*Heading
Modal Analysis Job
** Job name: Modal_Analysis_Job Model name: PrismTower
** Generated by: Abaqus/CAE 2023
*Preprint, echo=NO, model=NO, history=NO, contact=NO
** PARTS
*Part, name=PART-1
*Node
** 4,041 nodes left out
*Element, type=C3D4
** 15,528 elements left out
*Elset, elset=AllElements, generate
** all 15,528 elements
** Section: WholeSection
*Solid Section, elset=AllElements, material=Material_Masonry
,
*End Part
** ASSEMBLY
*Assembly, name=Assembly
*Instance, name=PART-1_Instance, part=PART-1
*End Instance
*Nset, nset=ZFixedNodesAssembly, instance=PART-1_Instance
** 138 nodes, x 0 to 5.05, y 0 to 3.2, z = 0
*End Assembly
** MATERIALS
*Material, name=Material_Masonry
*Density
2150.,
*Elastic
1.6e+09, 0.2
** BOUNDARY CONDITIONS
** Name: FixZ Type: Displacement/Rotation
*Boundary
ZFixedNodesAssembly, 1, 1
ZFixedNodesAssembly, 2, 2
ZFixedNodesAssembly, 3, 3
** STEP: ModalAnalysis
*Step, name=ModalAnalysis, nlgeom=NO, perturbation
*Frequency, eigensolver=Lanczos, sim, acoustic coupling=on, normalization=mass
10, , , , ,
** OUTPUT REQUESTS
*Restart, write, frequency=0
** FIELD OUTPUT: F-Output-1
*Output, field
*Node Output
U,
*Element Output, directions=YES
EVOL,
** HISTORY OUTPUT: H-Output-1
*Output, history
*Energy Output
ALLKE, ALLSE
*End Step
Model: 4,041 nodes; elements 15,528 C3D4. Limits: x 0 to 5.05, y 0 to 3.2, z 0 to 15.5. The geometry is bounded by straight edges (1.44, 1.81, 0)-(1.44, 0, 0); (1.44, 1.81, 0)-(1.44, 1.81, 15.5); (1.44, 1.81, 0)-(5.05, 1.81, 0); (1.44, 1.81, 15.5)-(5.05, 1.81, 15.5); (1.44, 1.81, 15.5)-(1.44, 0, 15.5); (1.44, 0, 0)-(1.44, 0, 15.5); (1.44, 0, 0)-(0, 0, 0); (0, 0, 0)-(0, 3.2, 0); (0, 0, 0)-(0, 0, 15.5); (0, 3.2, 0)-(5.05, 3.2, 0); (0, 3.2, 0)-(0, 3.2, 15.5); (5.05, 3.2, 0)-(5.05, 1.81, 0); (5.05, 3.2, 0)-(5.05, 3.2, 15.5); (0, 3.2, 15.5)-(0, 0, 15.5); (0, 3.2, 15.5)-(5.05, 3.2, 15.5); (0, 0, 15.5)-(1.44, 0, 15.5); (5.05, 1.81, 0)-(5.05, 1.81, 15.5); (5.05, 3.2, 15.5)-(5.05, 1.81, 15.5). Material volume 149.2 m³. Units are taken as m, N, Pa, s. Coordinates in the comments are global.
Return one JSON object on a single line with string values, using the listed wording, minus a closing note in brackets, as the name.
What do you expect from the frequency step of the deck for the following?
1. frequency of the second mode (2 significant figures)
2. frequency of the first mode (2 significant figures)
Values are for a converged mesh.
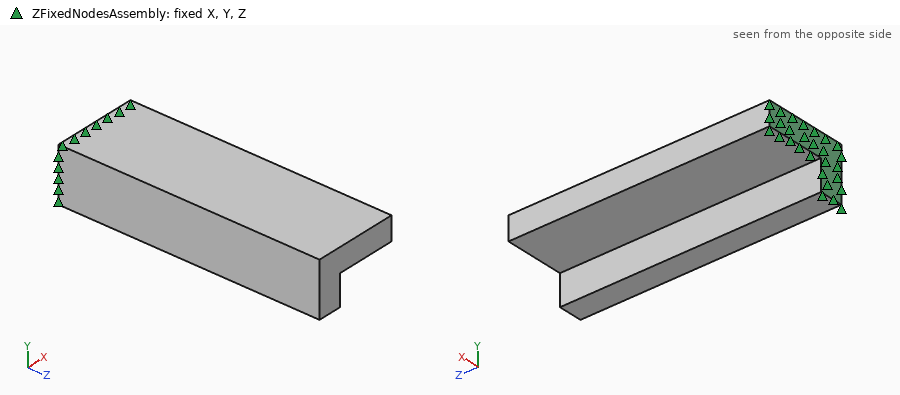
{"frequency of the second mode": "2.7 Hz", "frequency of the first mode": "1.4 Hz"}
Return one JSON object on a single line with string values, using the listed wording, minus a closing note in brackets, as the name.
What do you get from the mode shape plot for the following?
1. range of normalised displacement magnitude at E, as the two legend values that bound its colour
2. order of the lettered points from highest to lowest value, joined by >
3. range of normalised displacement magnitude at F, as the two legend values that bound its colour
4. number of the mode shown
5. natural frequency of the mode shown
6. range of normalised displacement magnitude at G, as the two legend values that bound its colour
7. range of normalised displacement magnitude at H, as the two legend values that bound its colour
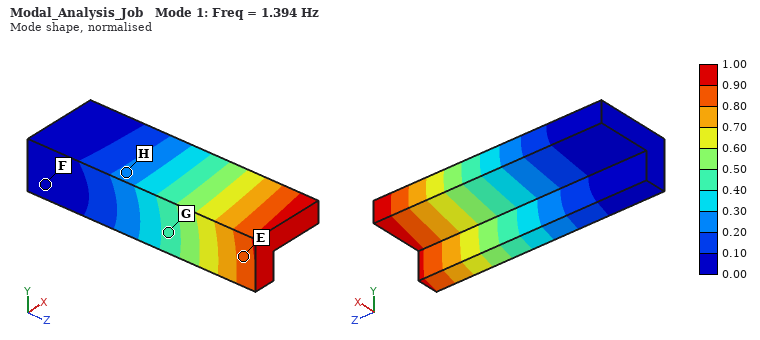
{"range of normalised displacement magnitude at E, as the two legend values that bound its colour": "0.80 to 0.90", "order of the lettered points from highest to lowest value, joined by >": "E > G > H > F", "range of normalised displacement magnitude at F, as the two legend values that bound its colour": "0.00 to 0.10", "number of the mode shown": "1", "natural frequency of the mode shown": "1.394 Hz", "range of normalised displacement magnitude at G, as the two legend values that bound its colour": "0.40 to 0.50", "range of normalised displacement magnitude at H, as the two legend values that bound its colour": "0.20 to 0.30"}
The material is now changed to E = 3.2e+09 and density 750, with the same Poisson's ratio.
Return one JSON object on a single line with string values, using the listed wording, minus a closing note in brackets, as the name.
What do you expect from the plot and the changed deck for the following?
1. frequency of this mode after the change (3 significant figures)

{"frequency of this mode after the change": "3.34 Hz"}
